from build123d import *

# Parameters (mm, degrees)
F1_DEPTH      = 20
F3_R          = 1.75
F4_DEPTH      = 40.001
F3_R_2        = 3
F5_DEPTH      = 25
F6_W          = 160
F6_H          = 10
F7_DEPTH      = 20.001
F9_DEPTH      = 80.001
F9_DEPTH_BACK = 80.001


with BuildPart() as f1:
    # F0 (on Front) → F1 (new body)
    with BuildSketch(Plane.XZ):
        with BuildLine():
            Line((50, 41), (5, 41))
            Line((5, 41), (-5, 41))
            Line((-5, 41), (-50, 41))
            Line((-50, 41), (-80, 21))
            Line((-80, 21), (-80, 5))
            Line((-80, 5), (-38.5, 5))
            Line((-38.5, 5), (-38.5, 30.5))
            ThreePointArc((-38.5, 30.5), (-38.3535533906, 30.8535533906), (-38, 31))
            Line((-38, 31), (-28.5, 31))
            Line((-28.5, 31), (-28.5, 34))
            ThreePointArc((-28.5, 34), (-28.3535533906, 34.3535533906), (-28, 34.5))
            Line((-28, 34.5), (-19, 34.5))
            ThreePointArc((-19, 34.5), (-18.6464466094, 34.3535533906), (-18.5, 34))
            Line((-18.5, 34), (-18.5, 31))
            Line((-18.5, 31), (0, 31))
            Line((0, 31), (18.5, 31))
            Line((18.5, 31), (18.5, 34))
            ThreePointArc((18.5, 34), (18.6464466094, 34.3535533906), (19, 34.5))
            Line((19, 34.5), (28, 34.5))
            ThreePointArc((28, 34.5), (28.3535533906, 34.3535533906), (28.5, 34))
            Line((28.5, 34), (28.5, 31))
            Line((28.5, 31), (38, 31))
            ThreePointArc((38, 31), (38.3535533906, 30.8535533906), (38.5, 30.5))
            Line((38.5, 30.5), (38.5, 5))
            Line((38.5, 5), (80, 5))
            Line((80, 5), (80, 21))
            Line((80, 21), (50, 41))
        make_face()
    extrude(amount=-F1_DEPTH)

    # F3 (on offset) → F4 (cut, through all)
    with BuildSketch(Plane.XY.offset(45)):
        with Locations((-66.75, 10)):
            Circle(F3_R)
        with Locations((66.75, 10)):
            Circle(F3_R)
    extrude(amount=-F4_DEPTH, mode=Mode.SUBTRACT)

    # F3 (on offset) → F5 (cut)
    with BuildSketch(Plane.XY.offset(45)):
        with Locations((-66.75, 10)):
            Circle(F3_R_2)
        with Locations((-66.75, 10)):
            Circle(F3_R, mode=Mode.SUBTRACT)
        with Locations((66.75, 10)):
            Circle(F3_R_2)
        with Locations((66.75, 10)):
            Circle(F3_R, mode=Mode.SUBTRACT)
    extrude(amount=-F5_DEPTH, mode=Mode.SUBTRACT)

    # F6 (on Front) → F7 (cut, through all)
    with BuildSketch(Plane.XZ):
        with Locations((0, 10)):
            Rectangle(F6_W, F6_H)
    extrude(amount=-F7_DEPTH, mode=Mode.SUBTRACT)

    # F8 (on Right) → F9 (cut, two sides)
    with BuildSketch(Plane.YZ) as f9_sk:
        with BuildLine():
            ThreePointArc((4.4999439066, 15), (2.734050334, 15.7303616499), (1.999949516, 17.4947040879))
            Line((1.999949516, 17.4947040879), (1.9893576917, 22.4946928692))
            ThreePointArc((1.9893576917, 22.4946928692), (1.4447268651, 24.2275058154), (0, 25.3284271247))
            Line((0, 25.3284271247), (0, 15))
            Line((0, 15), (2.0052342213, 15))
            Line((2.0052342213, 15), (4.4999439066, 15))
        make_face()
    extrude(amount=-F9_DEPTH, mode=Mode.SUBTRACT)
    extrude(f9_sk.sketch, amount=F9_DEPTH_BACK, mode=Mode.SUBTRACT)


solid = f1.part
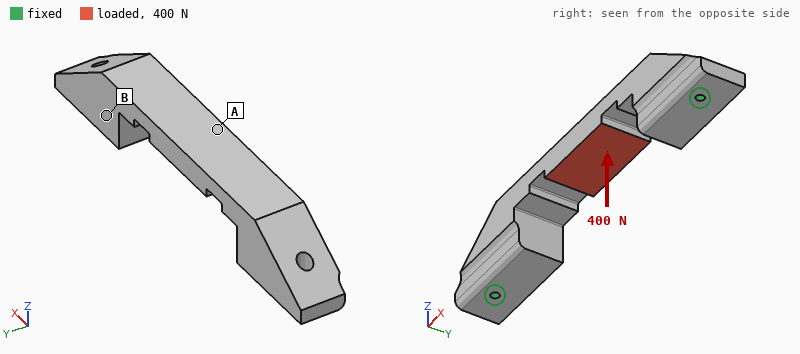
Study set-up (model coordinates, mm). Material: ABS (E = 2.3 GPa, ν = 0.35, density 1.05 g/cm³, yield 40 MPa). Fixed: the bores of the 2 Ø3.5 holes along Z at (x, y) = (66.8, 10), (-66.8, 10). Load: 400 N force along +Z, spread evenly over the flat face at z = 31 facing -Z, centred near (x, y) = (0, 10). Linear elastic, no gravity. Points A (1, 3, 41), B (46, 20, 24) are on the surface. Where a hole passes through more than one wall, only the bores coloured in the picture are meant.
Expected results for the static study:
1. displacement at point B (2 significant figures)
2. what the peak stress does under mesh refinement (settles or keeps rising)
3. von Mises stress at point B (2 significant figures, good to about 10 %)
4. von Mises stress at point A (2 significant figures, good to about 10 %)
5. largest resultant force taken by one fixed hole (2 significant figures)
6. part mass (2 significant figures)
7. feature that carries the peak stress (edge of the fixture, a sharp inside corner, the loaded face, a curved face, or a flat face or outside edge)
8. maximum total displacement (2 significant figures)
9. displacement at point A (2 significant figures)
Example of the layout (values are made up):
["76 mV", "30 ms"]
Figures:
["0.092 mm", "keeps rising", "2.3 MPa", "12 MPa", "450 N", "45 g", "edge of the fixture", "0.58 mm", "0.57 mm"]
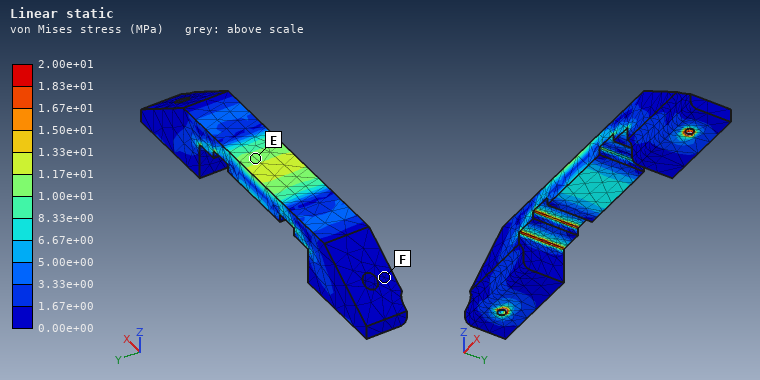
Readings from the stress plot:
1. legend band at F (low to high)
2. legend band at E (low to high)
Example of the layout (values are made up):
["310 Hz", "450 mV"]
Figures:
["0.00e+00 to 1.67e+00 MPa", "1.00e+01 to 1.17e+01 MPa"]
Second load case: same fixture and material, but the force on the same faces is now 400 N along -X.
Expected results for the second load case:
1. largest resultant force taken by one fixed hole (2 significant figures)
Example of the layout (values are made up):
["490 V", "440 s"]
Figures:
["200 N"]
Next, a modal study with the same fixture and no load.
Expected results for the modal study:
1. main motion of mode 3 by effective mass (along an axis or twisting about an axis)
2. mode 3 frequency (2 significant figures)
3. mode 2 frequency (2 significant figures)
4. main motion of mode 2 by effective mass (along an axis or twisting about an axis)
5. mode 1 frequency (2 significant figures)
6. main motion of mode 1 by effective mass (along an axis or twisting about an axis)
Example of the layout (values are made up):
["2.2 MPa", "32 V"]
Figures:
["along Z", "1400 Hz", "1000 Hz", "along X", "640 Hz", "along Y"]
